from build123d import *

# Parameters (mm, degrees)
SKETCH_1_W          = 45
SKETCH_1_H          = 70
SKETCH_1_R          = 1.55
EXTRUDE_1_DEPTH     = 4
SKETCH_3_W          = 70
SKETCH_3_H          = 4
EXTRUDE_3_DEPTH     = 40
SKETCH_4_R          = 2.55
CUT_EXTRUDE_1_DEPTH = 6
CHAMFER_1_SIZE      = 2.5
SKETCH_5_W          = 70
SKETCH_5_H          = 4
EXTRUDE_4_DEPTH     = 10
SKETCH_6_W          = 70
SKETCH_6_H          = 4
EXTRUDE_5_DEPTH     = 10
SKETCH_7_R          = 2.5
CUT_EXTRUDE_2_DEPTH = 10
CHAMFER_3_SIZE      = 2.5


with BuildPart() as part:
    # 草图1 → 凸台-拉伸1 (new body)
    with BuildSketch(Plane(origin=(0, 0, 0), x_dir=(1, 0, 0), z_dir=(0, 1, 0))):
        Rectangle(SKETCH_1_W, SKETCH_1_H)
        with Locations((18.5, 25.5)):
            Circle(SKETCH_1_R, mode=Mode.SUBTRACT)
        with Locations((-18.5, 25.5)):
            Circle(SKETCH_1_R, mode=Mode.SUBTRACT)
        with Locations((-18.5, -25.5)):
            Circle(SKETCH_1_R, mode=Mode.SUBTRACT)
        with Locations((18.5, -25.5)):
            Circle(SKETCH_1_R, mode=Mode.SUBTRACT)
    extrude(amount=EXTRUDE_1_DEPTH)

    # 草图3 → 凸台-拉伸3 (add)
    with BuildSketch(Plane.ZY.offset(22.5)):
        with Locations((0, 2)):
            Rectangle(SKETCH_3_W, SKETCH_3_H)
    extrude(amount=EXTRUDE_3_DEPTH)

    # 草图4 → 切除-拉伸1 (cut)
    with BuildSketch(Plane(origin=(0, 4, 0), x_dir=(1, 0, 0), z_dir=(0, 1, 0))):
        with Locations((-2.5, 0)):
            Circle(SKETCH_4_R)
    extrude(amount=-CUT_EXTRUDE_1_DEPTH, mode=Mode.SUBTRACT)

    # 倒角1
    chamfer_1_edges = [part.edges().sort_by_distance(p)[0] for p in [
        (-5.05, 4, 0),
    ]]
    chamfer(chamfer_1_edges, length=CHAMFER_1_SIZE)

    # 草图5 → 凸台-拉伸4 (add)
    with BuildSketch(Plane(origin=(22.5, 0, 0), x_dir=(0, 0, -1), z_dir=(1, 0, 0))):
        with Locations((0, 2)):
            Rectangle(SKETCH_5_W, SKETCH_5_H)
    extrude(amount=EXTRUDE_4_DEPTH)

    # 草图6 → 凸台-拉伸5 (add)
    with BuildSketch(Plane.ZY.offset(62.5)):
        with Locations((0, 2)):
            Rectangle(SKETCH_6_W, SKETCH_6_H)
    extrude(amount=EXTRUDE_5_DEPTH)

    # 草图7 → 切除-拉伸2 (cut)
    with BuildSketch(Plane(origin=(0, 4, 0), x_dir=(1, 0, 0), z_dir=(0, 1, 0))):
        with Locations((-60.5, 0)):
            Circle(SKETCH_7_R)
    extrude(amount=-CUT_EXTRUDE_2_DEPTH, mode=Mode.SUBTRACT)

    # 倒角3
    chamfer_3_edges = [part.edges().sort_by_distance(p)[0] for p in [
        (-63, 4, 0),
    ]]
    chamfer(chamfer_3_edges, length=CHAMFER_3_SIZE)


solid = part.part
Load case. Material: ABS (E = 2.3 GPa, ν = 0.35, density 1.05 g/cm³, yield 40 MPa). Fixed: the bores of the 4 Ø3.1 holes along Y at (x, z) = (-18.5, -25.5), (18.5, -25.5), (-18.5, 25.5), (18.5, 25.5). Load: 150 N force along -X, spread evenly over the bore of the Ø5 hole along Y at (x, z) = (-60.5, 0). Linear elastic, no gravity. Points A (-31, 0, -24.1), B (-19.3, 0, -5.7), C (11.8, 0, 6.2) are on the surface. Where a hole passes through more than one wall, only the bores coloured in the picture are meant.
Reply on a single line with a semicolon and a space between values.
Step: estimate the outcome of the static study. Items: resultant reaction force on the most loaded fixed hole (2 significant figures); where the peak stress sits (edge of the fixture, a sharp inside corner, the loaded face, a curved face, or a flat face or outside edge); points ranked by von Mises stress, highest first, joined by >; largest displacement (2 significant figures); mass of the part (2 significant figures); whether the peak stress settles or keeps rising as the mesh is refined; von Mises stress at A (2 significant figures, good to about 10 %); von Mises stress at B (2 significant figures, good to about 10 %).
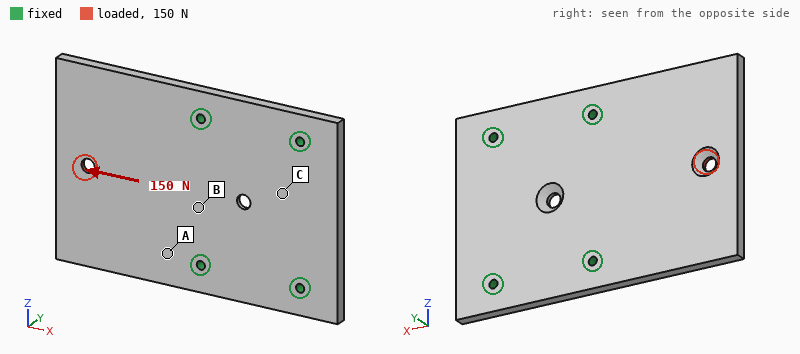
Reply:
58 N; a sharp inside corner; A > B > C; 0.36 mm; 30 g; keeps rising; 1.6 MPa; 1.00 MPa
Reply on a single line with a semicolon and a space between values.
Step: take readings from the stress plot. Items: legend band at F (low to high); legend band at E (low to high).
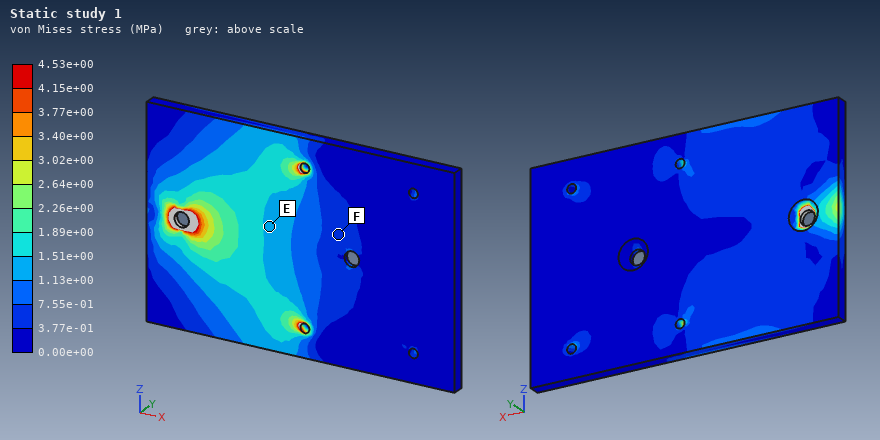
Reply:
3.77e-01 to 7.55e-01 MPa; 1.13e+00 to 1.51e+00 MPa
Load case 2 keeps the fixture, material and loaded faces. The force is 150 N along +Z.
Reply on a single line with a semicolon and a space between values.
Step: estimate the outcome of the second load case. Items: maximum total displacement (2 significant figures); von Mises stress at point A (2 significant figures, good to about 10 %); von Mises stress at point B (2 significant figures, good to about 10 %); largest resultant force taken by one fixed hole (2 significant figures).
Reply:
0.16 mm; 1.5 MPa; 0.73 MPa; 130 N
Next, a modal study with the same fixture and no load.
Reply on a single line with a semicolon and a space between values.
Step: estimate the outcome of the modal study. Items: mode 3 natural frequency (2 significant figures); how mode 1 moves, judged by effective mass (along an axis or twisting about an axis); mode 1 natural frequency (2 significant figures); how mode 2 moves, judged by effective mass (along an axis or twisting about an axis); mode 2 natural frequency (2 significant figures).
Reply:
1500 Hz; along Y; 300 Hz; twisting about X; 640 Hz
